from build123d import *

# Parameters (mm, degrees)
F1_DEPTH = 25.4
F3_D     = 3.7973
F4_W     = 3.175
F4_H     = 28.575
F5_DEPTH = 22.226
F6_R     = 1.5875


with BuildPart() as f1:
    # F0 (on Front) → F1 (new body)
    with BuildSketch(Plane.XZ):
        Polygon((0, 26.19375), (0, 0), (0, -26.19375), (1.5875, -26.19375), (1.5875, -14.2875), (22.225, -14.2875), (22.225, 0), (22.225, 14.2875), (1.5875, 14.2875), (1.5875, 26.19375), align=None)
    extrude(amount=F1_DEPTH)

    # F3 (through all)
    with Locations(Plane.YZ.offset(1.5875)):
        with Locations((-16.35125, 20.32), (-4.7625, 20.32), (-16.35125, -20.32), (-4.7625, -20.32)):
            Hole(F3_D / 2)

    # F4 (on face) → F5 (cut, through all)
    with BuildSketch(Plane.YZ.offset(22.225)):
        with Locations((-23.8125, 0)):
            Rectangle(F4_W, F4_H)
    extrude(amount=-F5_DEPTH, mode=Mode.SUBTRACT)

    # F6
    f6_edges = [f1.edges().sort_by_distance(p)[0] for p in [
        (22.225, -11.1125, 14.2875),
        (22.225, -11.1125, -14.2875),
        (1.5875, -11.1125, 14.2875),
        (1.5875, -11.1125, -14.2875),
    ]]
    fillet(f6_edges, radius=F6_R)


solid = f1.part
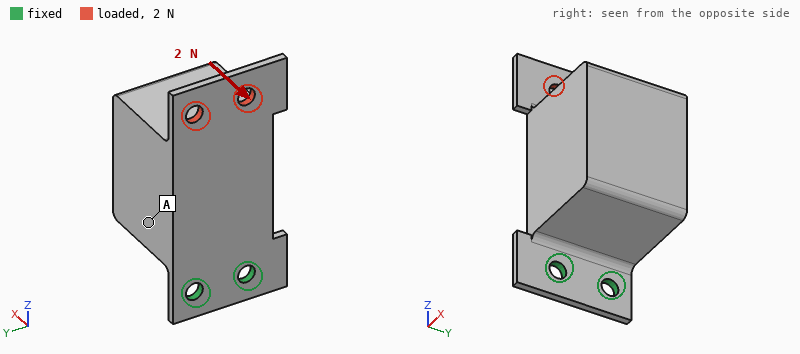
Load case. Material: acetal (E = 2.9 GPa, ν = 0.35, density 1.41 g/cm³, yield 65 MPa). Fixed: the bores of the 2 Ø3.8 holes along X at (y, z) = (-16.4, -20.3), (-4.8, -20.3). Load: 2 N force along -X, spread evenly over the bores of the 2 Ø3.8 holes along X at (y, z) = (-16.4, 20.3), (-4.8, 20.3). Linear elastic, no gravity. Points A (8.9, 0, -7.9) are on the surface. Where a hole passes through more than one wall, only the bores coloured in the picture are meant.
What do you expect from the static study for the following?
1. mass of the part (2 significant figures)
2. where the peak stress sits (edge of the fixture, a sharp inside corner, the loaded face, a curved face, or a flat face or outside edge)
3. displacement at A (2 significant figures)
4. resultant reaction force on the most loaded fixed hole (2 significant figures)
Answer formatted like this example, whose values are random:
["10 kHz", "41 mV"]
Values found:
["21 g", "a flat face or outside edge", "0.18 mm", "1.0 N"]
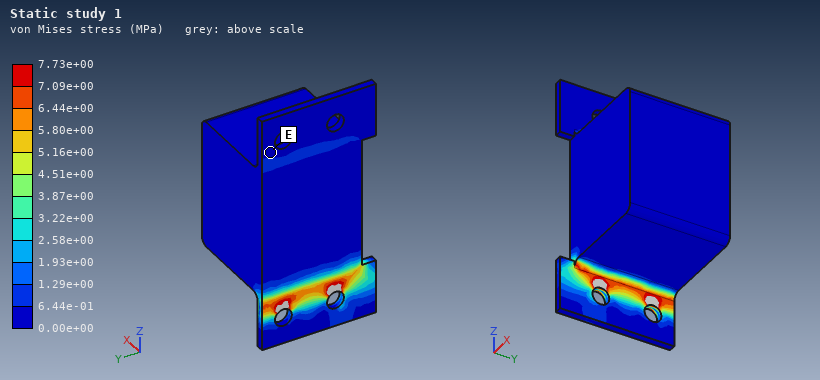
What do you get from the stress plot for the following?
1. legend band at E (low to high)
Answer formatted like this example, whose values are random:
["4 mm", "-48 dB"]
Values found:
["0.00e+00 to 6.44e-01 MPa"]
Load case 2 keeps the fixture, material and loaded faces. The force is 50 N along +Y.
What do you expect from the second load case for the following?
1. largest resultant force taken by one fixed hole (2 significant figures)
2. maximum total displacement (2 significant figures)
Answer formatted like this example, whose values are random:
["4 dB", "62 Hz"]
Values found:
["150 N", "0.28 mm"]
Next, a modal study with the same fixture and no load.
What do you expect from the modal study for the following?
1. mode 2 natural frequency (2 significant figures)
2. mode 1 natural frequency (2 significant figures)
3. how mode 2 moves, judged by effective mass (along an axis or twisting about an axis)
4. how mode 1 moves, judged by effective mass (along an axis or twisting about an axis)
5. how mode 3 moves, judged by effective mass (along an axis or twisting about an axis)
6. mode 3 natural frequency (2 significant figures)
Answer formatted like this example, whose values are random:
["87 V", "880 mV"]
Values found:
["600 Hz", "110 Hz", "along Y", "along X", "along Y", "1300 Hz"]
